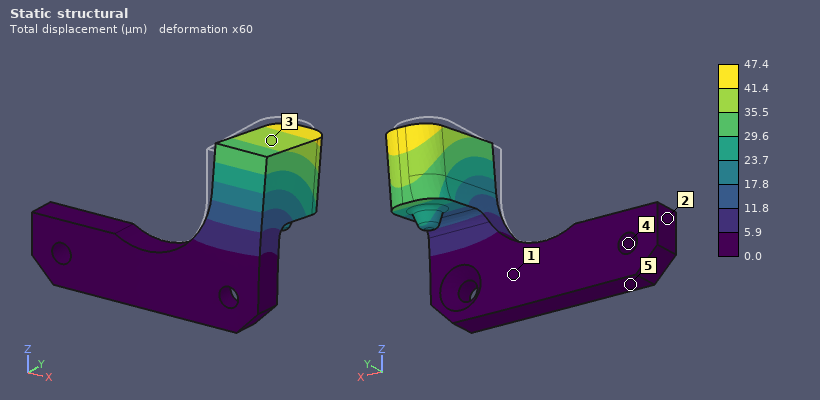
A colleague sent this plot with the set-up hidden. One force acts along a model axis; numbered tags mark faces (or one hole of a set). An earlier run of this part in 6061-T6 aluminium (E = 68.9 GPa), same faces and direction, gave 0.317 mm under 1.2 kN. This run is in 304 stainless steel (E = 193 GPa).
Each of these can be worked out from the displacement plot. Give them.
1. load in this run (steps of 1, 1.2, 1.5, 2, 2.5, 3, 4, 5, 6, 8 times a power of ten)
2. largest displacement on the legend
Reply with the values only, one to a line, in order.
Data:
500 N
47.4 µm
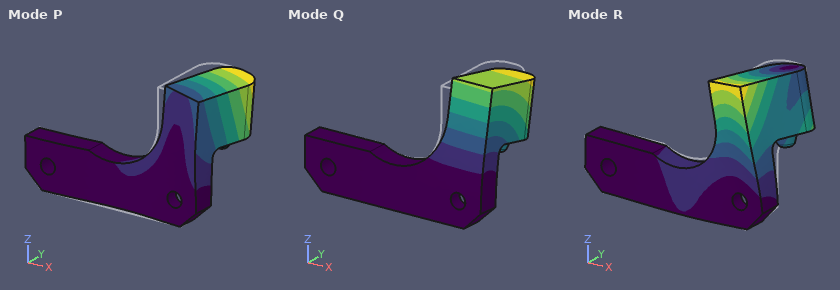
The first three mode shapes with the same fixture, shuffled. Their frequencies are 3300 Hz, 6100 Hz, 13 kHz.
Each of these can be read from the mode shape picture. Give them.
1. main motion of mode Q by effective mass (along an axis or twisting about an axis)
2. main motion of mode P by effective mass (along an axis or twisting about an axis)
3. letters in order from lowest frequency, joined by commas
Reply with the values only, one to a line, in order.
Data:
along Y
along X
Q, P, R
